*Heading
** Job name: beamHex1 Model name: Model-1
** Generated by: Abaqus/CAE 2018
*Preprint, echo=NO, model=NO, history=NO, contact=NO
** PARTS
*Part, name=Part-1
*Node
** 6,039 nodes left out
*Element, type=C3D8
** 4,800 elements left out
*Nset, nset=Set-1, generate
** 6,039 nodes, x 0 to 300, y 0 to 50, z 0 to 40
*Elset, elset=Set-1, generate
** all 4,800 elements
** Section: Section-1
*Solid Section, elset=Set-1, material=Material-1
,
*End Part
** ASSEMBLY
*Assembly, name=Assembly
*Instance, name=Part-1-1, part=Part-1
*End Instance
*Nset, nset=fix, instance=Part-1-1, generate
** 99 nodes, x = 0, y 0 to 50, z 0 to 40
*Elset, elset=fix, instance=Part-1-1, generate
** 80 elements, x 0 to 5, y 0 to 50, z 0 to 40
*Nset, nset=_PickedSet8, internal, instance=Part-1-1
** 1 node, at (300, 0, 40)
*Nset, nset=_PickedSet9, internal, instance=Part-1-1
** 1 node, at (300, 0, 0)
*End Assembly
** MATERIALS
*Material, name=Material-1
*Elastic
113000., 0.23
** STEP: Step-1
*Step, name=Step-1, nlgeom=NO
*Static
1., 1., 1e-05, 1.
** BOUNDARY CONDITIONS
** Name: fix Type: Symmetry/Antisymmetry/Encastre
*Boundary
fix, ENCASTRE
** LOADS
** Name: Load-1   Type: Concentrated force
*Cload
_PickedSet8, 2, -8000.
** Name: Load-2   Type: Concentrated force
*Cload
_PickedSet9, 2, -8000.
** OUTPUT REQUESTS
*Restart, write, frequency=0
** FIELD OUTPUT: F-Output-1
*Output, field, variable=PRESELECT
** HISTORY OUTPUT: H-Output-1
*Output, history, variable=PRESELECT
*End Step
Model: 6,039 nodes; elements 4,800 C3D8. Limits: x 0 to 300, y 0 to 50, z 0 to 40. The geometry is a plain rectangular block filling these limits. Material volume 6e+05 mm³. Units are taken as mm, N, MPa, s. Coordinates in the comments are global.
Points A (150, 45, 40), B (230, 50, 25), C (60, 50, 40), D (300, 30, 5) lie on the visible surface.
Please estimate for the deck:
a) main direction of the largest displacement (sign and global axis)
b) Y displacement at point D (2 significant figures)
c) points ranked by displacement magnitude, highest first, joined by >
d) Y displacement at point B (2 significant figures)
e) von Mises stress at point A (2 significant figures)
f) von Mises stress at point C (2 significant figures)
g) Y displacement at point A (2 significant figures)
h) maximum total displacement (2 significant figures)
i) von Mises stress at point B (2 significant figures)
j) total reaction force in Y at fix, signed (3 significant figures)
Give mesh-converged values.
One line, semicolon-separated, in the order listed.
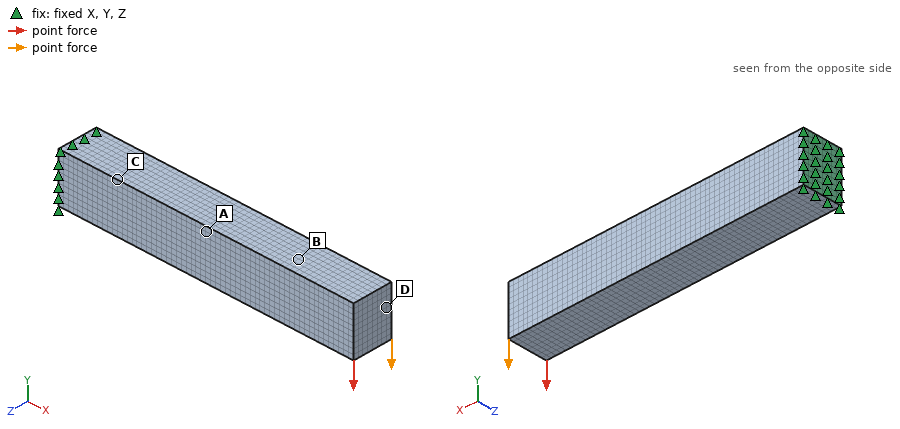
-Y; -3.1 mm; D > B > A > C; -2.0 mm; 120 MPa; 230 MPa; -0.98 mm; 3.4 mm; 67 MPa; 16000 N
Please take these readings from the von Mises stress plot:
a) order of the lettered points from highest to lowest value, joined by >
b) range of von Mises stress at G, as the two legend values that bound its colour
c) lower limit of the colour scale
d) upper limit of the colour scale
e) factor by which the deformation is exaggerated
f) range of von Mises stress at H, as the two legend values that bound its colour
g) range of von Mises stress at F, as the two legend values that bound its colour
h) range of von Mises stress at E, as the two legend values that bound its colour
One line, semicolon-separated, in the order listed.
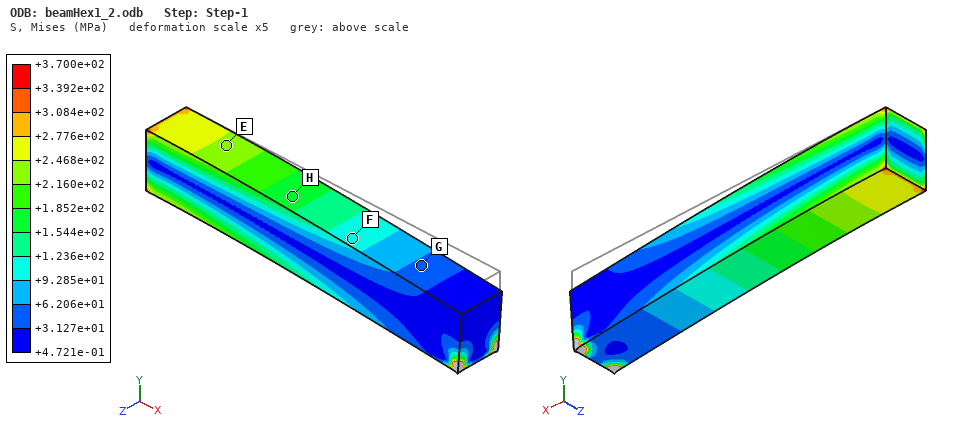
E > H > F > G; +3.127e+01 to +6.206e+01 MPa; +4.721e-01 MPa; +3.700e+02 MPa; 5; +1.544e+02 to +1.852e+02 MPa; +9.285e+01 to +1.236e+02 MPa; +2.160e+02 to +2.468e+02 MPa
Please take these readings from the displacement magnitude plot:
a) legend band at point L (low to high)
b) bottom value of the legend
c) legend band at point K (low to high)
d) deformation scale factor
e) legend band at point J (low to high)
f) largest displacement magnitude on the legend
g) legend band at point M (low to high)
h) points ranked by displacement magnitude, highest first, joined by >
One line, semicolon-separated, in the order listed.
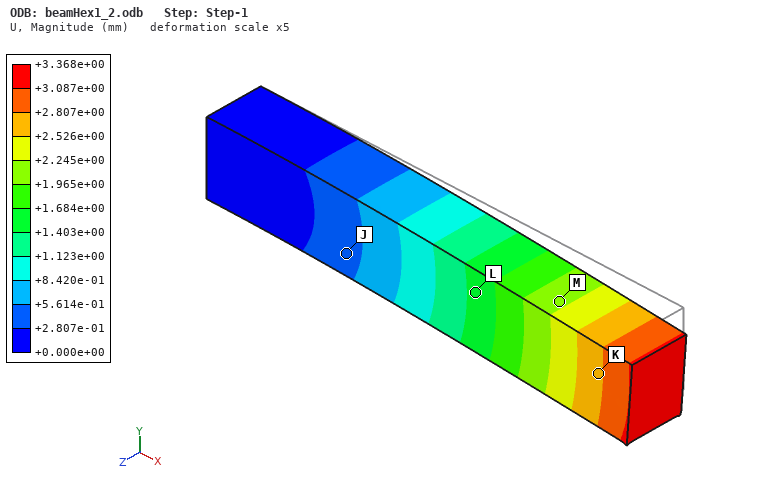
+1.403e+00 to +1.684e+00 mm; +0.000e+00 mm; +2.526e+00 to +2.807e+00 mm; 5; +2.807e-01 to +5.614e-01 mm; +3.368e+00 mm; +1.965e+00 to +2.245e+00 mm; K > M > L > J
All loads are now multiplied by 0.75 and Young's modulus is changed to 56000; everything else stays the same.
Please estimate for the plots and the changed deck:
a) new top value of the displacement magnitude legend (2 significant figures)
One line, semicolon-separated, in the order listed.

5.1 mm
